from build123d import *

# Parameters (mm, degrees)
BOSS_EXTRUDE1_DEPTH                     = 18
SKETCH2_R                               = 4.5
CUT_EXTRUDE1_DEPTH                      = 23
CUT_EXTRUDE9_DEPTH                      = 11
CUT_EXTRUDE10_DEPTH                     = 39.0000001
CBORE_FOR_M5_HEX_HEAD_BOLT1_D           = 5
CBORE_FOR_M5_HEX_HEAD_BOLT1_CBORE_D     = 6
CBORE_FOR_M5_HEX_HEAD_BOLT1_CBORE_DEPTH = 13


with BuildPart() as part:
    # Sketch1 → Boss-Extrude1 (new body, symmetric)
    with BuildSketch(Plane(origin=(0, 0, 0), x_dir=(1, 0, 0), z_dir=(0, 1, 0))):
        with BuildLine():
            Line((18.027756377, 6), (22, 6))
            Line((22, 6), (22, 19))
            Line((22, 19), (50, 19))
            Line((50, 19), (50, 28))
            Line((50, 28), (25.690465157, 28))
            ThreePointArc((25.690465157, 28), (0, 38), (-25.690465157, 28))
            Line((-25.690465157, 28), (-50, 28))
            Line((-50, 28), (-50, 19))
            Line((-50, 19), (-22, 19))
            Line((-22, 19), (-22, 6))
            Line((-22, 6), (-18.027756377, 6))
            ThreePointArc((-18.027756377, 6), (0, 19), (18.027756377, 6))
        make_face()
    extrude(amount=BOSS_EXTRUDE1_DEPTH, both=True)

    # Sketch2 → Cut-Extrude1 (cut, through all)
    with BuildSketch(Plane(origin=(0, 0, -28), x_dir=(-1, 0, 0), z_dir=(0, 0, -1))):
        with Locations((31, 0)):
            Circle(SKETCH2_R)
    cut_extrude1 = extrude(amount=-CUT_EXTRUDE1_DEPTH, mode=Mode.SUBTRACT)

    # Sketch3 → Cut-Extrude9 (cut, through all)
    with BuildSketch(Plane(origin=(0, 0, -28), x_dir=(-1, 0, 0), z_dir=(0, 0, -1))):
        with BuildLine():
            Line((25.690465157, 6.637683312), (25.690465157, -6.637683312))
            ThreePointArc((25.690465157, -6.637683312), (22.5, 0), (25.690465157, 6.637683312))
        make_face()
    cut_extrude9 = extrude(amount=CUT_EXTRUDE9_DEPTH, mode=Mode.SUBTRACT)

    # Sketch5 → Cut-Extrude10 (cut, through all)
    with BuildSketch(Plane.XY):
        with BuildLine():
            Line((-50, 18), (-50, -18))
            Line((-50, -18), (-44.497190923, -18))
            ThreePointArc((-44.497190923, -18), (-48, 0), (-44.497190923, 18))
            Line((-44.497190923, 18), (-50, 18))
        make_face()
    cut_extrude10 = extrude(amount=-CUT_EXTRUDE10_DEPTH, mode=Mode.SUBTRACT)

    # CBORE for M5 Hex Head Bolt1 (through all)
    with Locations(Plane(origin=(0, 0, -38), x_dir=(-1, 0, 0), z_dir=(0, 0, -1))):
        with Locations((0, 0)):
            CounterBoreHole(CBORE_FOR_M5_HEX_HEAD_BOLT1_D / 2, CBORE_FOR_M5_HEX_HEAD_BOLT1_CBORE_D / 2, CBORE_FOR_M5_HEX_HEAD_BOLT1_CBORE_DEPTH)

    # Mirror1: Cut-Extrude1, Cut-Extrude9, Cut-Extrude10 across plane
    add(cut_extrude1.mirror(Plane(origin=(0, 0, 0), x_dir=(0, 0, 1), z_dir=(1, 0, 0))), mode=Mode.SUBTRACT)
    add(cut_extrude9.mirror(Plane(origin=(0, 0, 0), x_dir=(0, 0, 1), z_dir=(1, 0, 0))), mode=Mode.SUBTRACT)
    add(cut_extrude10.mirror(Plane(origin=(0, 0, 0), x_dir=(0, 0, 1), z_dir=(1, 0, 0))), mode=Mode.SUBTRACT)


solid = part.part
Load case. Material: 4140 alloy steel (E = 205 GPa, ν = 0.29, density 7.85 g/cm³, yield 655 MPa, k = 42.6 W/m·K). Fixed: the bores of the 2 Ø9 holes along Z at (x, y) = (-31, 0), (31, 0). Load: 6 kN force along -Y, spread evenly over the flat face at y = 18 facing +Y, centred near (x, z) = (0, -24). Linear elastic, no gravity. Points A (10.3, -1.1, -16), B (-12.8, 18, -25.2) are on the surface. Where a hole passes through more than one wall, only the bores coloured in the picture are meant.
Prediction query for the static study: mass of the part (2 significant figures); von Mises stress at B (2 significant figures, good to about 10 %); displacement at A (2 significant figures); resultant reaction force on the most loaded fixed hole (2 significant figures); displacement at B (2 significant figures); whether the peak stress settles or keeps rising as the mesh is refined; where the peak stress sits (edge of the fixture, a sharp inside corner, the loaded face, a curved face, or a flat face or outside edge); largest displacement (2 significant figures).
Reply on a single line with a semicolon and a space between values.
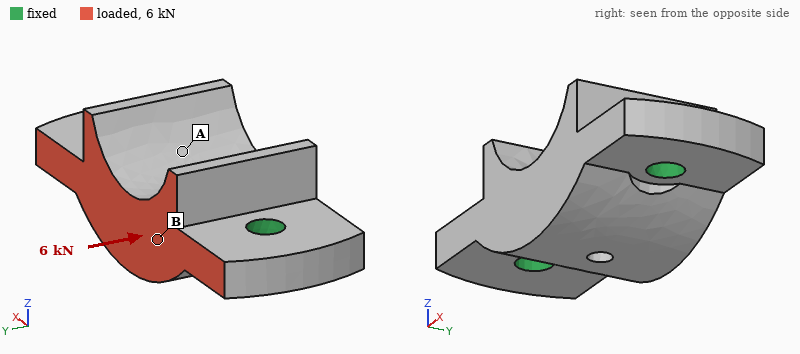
390 g; 8.8 MPa; 1.5 µm; 3.0 kN; 2.1 µm; keeps rising; edge of the fixture; 3.0 µm
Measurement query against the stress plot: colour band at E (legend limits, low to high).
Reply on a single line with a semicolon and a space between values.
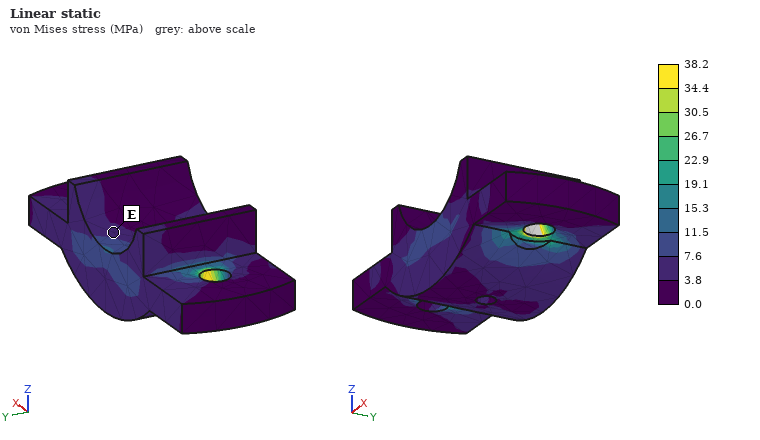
3.8 to 7.6 MPa
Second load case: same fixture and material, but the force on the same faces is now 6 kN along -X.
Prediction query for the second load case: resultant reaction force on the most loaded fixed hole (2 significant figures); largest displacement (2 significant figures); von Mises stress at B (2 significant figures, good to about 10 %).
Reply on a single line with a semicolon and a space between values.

3.4 kN; 3.3 µm; 7.9 MPa
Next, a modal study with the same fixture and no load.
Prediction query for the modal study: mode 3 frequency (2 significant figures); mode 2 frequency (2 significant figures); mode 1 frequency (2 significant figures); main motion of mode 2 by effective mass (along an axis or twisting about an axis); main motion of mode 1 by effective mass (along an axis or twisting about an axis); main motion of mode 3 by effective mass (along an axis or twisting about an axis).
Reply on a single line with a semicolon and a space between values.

15 kHz; 12 kHz; 9100 Hz; along Z; twisting about X; along Y
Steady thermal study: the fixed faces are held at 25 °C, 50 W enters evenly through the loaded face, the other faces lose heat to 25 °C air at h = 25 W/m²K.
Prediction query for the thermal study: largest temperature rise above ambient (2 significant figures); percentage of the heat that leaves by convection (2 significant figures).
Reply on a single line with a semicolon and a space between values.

31 K; 7.0 %
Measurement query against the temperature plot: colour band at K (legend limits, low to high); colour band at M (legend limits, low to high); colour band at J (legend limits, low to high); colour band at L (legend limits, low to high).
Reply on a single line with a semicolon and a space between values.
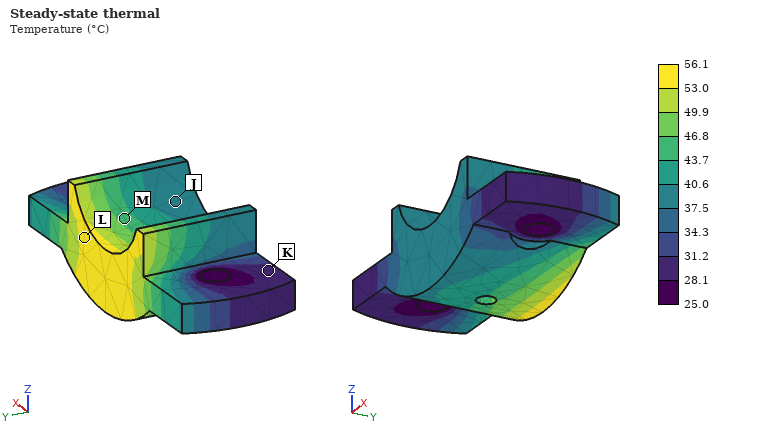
28.1 to 31.2 °C; 43.7 to 46.8 °C; 37.5 to 40.6 °C; 53.0 to 56.1 °C
